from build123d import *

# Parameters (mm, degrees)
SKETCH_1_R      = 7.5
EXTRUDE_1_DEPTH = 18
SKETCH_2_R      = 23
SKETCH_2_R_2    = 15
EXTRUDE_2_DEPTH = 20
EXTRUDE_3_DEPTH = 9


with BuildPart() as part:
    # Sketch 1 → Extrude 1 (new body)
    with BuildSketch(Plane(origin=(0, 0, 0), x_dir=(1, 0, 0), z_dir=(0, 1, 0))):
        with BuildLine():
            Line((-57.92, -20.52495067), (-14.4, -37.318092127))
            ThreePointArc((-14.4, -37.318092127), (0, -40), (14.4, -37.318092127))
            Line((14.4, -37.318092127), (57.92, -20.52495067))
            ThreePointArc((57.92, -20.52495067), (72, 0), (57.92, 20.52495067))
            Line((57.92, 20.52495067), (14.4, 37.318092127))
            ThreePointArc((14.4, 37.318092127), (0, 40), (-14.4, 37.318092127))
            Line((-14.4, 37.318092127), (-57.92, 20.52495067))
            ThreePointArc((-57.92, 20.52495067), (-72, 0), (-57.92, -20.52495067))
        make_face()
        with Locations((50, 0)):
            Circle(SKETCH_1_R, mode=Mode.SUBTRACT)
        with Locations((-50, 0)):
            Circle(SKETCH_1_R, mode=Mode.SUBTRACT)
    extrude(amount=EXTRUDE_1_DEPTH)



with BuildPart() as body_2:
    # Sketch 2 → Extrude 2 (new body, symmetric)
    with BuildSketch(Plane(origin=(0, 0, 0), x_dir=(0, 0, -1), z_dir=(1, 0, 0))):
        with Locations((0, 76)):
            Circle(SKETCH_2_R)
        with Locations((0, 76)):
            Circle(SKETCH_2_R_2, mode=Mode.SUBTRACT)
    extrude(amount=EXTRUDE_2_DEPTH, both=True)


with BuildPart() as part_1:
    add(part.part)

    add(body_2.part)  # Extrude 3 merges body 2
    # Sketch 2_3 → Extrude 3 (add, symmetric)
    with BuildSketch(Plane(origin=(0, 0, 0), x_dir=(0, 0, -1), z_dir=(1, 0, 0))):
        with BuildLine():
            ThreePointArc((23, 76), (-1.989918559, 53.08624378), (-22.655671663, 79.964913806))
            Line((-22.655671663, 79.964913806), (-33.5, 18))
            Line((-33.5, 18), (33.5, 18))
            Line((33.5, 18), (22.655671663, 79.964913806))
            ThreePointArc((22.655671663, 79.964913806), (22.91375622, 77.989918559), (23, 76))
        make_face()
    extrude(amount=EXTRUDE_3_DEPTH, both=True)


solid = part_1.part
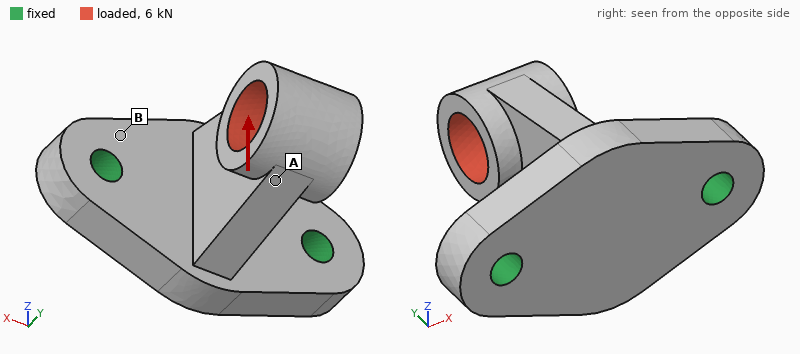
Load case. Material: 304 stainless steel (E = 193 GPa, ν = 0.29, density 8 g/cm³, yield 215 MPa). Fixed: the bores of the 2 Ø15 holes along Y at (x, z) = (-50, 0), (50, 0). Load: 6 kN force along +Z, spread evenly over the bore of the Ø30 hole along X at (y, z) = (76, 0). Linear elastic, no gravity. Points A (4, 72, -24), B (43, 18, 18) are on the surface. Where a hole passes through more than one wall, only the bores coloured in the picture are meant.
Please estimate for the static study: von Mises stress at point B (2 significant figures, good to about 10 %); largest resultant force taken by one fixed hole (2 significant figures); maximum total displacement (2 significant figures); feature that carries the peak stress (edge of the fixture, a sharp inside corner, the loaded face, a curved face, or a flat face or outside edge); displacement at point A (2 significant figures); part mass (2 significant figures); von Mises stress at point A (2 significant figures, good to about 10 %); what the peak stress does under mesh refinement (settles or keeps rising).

48 MPa
3.0 kN
0.10 mm
edge of the fixture
0.076 mm
1.8 kg
21 MPa
keeps rising
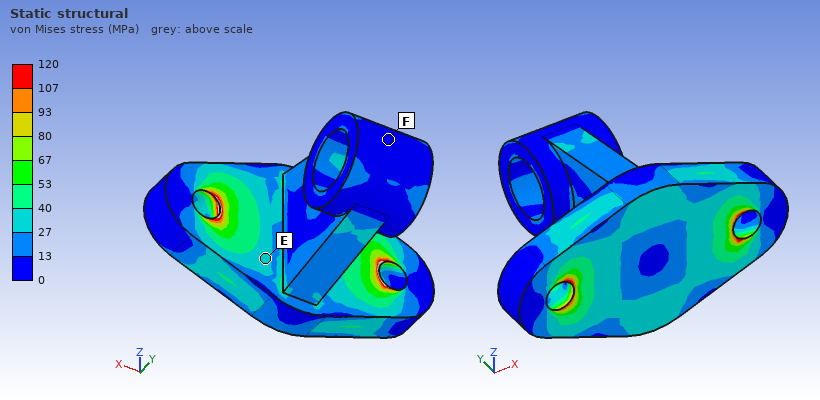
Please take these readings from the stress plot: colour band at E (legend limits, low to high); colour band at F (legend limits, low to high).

27 to 40 MPa
0 to 13 MPa
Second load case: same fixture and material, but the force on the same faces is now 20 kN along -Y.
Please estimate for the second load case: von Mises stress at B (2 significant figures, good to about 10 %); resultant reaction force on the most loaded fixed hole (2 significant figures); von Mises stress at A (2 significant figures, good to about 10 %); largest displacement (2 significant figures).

27 MPa
10 kN
18 MPa
32 µm
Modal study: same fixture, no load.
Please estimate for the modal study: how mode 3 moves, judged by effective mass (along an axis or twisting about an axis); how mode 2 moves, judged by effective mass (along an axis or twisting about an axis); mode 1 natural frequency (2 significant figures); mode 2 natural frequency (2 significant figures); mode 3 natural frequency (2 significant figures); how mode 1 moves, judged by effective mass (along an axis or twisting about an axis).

along Y
along Z
1900 Hz
2100 Hz
4600 Hz
along X
